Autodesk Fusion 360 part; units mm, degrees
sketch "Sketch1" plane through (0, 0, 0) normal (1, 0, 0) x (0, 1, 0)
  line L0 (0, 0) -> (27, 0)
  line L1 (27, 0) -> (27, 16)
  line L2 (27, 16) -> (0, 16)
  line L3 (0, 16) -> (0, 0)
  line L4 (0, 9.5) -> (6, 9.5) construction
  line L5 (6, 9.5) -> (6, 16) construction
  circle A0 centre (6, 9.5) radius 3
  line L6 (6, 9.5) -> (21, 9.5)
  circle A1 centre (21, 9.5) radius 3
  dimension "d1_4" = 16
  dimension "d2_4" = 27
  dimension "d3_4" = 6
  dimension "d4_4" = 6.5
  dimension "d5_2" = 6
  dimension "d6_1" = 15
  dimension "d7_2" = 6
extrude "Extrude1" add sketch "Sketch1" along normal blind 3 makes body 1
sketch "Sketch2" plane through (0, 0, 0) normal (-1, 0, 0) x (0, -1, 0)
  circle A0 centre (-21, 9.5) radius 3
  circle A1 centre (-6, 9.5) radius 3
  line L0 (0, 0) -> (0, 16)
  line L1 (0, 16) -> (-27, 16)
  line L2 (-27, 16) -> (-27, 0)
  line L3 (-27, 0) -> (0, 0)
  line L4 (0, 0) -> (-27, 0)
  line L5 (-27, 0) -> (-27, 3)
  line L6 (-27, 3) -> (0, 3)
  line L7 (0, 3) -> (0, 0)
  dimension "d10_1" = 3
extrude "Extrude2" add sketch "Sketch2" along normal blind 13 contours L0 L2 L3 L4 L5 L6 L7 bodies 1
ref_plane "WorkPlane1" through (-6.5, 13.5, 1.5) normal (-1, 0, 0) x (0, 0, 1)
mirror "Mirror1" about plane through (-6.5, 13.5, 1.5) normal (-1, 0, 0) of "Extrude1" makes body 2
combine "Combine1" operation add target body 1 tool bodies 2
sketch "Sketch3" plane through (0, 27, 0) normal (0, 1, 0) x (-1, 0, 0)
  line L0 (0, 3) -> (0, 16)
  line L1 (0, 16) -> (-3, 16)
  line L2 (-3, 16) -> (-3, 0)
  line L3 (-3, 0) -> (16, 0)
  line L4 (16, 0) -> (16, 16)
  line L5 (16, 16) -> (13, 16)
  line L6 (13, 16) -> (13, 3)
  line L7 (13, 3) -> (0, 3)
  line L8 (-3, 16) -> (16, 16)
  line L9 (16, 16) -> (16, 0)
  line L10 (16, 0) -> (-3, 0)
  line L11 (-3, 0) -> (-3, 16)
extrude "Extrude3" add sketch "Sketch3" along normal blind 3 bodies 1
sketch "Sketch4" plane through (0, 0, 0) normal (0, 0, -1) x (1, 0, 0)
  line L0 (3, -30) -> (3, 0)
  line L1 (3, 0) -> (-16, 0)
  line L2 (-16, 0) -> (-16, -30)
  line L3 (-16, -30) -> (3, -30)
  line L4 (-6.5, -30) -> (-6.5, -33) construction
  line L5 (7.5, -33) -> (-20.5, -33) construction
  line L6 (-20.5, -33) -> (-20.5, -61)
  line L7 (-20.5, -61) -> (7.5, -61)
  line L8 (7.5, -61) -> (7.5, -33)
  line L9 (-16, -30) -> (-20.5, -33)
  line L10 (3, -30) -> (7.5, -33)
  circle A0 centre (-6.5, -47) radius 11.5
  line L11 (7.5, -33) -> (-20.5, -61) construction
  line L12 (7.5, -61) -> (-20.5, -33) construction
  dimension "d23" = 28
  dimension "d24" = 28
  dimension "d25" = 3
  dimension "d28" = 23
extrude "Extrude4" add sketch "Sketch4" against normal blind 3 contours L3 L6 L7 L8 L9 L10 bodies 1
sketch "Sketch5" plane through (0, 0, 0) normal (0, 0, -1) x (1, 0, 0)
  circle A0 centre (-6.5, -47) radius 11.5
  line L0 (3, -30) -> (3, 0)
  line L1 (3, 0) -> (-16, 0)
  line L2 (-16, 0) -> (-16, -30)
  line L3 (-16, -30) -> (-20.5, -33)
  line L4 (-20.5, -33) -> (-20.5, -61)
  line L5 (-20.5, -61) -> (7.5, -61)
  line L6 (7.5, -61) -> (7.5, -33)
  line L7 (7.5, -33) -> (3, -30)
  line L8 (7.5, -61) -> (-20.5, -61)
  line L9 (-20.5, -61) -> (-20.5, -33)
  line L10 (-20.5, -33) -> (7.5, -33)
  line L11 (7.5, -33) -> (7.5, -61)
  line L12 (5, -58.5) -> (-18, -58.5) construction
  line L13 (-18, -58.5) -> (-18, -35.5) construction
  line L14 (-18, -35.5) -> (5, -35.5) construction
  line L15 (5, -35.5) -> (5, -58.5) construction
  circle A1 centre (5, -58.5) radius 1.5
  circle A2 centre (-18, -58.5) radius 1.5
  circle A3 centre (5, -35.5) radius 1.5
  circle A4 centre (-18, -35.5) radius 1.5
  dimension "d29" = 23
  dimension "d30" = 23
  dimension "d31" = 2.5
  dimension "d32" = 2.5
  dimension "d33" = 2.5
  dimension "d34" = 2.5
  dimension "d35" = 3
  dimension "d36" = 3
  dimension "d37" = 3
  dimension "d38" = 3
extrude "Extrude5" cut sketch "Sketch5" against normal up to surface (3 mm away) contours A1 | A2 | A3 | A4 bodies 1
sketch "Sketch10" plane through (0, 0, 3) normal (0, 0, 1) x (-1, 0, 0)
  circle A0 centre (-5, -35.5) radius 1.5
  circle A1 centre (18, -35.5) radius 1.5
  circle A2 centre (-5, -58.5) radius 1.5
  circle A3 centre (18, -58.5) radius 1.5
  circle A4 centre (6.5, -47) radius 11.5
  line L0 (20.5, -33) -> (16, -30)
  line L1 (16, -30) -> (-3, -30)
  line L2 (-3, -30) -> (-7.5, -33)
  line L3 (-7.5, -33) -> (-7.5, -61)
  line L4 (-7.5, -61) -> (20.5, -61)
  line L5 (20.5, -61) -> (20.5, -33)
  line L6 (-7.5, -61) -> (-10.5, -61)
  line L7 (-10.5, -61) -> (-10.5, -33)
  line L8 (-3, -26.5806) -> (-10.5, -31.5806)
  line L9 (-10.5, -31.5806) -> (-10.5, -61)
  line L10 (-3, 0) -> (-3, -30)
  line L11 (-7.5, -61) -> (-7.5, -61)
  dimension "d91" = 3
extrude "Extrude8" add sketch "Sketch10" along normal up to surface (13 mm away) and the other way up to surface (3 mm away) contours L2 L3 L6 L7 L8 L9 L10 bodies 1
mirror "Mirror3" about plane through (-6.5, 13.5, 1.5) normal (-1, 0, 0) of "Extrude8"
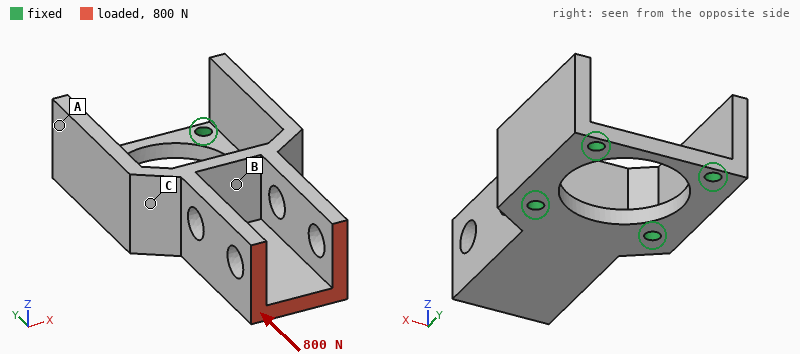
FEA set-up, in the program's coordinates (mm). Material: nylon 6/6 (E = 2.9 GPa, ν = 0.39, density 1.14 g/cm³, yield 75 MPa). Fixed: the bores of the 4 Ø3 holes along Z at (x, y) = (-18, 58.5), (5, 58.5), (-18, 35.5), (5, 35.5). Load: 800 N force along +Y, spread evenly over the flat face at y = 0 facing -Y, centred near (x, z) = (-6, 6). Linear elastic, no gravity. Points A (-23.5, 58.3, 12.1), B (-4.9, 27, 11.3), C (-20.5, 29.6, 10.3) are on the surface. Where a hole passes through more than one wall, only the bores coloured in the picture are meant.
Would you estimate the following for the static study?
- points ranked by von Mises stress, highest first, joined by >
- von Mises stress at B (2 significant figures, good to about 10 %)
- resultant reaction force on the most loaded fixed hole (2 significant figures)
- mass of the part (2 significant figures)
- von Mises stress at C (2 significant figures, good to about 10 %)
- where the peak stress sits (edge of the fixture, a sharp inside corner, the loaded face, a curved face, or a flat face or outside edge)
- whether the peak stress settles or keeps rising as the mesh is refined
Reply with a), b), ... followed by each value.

a) C > B > A
b) 8.3 MPa
c) 390 N
d) 10 g
e) 13 MPa
f) edge of the fixture
g) keeps rising
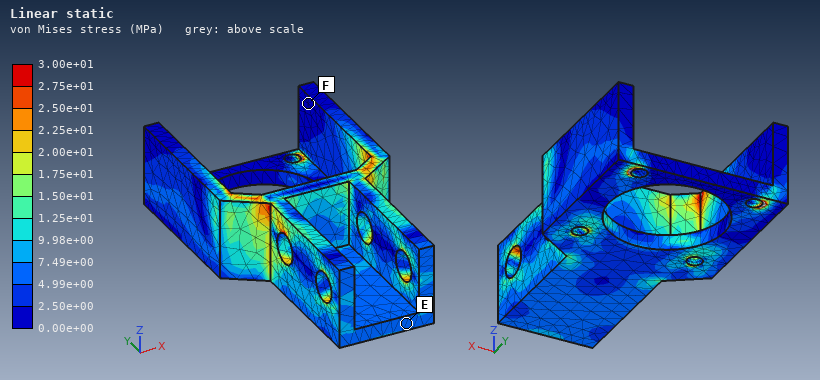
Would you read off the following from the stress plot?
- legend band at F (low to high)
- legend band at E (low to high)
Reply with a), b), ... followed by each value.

a) 0.00e+00 to 2.50e+00 MPa
b) 4.99e+00 to 7.49e+00 MPa
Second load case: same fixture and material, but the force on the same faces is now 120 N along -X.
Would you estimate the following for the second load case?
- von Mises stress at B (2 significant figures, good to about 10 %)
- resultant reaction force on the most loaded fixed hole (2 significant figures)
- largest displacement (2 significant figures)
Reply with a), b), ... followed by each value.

a) 3.4 MPa
b) 180 N
c) 0.80 mm
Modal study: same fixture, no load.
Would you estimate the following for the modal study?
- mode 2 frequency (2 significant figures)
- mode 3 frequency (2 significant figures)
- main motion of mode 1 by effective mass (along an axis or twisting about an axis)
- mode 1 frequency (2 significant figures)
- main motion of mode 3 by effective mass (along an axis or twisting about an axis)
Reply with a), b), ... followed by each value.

a) 2000 Hz
b) 3100 Hz
c) along Z
d) 1300 Hz
e) along X
